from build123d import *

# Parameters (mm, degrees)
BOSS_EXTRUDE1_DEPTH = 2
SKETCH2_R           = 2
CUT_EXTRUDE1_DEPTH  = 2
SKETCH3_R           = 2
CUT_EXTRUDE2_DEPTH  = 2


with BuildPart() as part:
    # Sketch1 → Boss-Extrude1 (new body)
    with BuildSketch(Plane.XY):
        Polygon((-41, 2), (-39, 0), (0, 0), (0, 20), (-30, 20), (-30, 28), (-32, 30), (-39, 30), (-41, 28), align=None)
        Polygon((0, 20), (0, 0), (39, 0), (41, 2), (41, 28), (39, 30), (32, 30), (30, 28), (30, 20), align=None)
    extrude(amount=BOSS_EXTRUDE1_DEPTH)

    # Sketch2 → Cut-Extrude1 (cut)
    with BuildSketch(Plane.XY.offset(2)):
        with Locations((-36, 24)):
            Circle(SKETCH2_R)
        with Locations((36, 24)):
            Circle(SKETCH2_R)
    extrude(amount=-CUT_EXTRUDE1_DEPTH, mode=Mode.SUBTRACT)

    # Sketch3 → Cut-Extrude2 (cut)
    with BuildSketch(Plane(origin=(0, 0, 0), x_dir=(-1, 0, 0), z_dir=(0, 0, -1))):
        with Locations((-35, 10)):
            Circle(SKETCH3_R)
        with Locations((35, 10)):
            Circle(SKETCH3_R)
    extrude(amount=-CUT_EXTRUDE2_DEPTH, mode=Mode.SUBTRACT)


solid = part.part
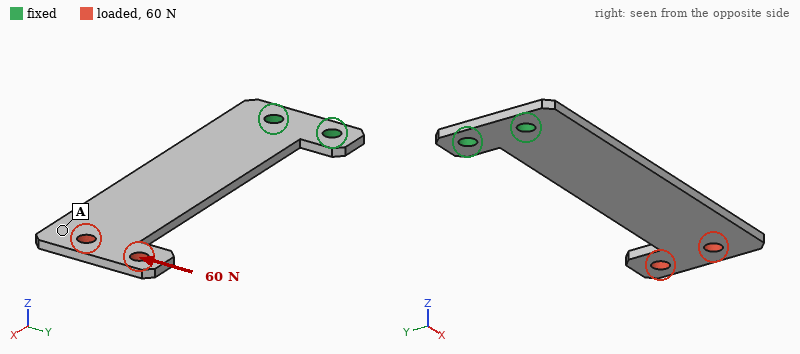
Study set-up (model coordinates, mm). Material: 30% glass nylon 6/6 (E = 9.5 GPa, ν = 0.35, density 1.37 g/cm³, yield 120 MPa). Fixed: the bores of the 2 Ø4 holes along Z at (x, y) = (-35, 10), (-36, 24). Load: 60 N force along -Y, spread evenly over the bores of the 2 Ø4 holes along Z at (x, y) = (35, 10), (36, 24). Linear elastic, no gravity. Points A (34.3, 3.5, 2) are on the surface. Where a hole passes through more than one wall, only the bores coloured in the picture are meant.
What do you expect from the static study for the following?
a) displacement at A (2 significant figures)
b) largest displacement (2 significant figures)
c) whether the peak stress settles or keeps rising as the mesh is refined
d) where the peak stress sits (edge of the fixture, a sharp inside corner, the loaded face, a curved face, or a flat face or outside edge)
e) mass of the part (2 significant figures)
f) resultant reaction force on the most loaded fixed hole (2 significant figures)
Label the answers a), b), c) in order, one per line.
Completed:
a) 0.73 mm
b) 0.86 mm
c) keeps rising
d) a sharp inside corner
e) 4.9 g
f) 260 N
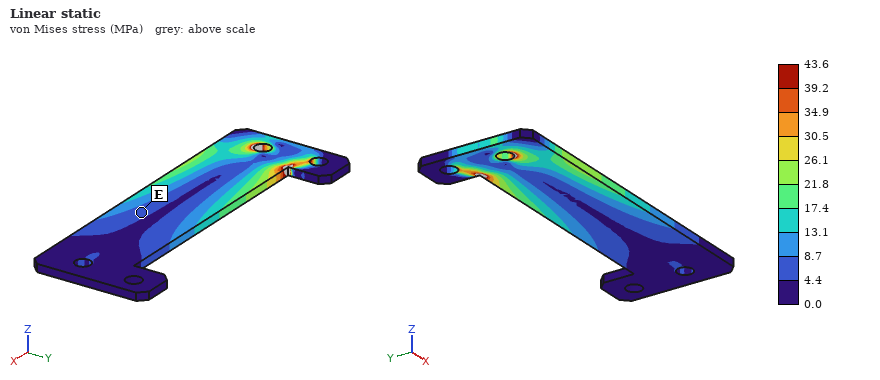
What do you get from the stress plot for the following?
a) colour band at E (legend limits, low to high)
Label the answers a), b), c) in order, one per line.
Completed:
a) 4.4 to 8.7 MPa
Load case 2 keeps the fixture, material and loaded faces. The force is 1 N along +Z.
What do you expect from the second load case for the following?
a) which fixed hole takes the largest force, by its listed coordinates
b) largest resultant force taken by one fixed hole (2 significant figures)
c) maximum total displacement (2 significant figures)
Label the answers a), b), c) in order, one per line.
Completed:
a) (-35, 10)
b) 1.7 N
c) 1.0 mm
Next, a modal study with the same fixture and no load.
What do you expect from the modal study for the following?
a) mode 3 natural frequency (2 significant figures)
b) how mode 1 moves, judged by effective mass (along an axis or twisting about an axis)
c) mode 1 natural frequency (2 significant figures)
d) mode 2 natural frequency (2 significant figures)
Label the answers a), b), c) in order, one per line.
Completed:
a) 980 Hz
b) along Z
c) 140 Hz
d) 760 Hz
